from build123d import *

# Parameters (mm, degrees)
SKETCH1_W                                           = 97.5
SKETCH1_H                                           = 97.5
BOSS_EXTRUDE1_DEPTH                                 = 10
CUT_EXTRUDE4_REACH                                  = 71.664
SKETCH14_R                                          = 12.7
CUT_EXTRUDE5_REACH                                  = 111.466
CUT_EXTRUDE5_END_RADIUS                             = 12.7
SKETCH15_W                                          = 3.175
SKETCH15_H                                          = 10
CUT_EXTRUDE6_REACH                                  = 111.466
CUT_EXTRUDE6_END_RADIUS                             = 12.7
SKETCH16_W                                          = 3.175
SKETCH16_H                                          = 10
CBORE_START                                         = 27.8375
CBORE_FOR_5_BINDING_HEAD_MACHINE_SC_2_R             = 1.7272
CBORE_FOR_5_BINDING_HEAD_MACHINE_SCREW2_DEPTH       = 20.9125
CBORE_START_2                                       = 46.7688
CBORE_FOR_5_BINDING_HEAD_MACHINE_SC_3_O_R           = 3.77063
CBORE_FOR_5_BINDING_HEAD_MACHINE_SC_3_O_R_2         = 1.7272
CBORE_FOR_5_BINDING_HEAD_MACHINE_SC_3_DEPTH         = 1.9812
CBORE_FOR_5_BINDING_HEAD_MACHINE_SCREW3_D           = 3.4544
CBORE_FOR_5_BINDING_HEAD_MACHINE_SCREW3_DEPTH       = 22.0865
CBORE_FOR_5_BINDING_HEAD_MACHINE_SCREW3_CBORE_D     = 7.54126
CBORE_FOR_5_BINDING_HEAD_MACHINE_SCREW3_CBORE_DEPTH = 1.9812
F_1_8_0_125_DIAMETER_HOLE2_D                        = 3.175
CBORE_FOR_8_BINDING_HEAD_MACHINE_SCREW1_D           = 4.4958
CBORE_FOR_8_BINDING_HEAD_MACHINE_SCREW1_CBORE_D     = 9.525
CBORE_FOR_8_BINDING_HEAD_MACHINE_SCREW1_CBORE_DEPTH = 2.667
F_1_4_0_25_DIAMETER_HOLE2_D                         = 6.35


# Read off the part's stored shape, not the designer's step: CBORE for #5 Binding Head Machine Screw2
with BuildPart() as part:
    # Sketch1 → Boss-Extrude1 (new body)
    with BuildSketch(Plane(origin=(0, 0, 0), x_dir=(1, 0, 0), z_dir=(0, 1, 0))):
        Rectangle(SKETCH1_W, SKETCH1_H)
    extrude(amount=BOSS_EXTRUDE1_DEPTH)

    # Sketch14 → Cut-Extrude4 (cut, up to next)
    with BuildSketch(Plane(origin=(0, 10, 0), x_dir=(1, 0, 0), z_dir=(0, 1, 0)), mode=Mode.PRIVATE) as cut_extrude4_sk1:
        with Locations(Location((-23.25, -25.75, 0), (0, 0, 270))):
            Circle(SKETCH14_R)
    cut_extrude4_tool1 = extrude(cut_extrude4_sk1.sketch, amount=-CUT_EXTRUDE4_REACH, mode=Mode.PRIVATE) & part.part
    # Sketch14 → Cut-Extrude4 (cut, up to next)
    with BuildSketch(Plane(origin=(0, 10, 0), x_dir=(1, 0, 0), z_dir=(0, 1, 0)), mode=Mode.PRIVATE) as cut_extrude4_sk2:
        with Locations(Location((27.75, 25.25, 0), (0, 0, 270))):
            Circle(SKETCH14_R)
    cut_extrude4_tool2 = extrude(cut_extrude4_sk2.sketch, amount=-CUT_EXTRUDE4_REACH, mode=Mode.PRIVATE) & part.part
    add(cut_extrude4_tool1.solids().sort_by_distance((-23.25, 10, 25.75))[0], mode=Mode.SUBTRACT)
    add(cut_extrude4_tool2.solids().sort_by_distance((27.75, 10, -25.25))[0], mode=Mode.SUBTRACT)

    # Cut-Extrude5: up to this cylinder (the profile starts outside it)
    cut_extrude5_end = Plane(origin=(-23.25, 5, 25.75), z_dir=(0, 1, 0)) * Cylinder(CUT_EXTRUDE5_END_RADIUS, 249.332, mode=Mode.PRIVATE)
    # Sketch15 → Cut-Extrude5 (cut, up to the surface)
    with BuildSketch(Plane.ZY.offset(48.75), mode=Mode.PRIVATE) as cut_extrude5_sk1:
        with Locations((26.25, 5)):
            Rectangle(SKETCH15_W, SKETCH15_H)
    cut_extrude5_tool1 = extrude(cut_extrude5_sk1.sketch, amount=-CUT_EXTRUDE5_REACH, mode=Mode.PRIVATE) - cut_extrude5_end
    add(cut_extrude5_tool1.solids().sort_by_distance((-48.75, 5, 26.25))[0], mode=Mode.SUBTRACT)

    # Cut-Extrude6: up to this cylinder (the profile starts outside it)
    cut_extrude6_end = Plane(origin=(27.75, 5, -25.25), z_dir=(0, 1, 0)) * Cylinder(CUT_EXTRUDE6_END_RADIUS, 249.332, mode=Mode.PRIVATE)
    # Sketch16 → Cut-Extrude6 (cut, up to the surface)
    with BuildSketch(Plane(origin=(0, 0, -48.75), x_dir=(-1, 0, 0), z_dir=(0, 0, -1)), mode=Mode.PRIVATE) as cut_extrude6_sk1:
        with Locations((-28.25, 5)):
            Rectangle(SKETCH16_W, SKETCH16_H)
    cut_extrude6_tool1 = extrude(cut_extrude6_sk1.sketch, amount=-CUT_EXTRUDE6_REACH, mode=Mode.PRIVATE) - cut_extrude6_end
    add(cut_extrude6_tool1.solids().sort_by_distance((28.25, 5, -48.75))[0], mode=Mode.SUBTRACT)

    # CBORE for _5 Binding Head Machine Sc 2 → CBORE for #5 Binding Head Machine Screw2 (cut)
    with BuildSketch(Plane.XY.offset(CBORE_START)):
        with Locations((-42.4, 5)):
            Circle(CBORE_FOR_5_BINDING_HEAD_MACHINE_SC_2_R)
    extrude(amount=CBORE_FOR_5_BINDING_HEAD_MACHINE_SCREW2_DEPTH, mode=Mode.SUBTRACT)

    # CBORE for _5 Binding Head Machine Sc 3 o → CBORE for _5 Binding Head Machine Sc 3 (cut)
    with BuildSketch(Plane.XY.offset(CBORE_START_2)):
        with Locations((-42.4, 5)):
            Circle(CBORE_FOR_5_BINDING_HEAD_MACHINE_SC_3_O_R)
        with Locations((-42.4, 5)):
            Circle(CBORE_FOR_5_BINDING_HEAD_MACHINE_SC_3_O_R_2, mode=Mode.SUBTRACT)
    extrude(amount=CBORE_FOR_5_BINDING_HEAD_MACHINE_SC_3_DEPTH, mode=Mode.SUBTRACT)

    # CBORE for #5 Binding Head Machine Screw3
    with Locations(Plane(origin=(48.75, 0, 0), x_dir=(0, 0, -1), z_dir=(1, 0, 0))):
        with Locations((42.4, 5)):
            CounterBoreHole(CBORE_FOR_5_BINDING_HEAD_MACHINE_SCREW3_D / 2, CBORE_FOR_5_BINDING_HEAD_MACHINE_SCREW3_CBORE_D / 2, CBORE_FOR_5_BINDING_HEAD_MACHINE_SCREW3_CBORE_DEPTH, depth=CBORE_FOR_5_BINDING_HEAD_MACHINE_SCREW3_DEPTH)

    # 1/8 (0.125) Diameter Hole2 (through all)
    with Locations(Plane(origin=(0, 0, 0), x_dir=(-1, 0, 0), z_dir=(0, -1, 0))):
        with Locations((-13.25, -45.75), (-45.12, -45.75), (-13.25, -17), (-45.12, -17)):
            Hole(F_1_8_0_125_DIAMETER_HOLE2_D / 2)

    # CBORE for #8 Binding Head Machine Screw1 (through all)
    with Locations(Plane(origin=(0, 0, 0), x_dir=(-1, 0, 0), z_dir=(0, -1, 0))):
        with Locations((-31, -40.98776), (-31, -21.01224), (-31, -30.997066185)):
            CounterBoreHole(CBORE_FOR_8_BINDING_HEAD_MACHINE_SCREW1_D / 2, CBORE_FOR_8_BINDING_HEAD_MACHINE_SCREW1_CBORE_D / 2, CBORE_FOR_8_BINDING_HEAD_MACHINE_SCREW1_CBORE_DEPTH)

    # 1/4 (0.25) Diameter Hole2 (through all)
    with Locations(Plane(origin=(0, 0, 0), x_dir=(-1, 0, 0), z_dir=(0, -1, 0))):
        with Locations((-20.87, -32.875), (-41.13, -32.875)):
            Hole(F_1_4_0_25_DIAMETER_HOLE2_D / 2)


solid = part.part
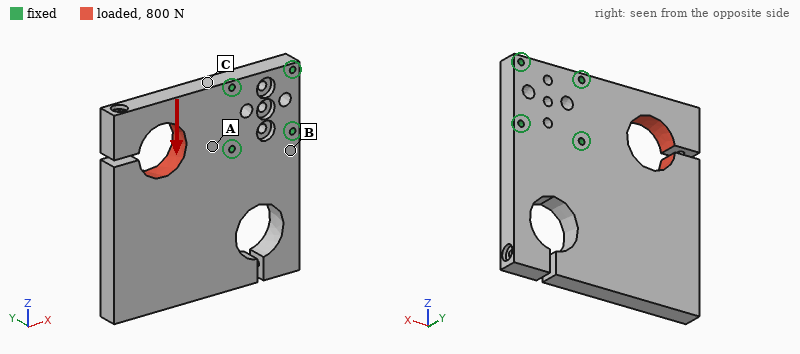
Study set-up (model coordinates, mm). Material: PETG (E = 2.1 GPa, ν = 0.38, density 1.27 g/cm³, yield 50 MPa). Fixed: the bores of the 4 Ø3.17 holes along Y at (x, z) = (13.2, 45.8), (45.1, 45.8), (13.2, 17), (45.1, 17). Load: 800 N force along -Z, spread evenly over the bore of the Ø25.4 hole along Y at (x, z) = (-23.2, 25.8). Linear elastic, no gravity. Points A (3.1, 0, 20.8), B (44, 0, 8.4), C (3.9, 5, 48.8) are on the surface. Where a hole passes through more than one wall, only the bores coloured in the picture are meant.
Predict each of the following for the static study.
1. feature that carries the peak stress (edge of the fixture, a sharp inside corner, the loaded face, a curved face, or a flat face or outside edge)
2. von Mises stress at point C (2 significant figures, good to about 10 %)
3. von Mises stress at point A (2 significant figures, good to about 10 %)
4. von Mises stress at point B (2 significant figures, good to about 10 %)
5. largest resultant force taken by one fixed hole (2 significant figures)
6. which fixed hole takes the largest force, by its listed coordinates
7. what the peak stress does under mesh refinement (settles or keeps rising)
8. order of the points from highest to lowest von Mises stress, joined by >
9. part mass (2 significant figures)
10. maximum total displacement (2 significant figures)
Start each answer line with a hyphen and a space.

- edge of the fixture
- 7.9 MPa
- 5.2 MPa
- 2.3 MPa
- 890 N
- (13.2, 17)
- keeps rising
- C > A > B
- 100 g
- 0.95 mm
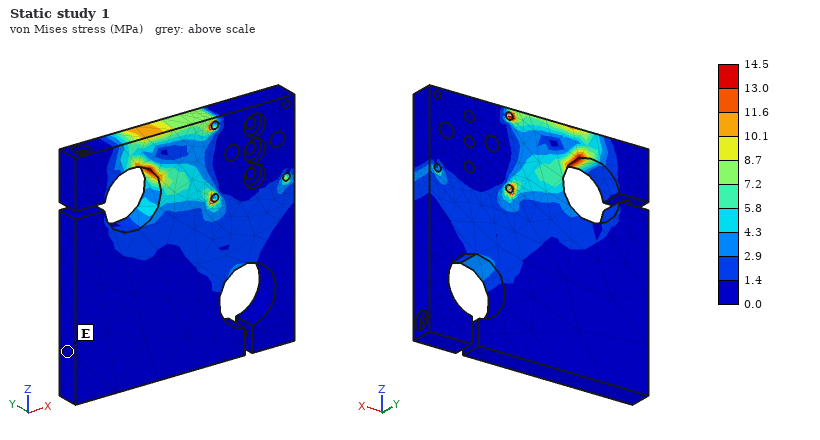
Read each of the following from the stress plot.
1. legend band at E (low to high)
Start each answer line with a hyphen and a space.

- 0.0 to 1.4 MPa
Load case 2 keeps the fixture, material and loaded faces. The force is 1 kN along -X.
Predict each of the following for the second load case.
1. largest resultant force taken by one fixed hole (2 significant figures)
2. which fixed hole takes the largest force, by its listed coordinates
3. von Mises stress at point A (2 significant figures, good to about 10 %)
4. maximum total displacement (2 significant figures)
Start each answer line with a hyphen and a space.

- 560 N
- (13.2, 17)
- 2.8 MPa
- 0.69 mm
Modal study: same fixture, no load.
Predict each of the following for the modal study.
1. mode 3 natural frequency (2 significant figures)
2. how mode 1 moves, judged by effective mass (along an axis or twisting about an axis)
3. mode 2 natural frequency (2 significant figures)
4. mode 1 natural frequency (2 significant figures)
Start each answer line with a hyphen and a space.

- 610 Hz
- along Y
- 480 Hz
- 280 Hz
